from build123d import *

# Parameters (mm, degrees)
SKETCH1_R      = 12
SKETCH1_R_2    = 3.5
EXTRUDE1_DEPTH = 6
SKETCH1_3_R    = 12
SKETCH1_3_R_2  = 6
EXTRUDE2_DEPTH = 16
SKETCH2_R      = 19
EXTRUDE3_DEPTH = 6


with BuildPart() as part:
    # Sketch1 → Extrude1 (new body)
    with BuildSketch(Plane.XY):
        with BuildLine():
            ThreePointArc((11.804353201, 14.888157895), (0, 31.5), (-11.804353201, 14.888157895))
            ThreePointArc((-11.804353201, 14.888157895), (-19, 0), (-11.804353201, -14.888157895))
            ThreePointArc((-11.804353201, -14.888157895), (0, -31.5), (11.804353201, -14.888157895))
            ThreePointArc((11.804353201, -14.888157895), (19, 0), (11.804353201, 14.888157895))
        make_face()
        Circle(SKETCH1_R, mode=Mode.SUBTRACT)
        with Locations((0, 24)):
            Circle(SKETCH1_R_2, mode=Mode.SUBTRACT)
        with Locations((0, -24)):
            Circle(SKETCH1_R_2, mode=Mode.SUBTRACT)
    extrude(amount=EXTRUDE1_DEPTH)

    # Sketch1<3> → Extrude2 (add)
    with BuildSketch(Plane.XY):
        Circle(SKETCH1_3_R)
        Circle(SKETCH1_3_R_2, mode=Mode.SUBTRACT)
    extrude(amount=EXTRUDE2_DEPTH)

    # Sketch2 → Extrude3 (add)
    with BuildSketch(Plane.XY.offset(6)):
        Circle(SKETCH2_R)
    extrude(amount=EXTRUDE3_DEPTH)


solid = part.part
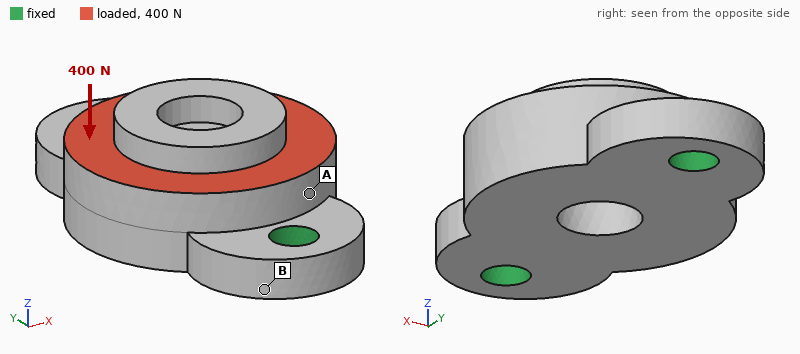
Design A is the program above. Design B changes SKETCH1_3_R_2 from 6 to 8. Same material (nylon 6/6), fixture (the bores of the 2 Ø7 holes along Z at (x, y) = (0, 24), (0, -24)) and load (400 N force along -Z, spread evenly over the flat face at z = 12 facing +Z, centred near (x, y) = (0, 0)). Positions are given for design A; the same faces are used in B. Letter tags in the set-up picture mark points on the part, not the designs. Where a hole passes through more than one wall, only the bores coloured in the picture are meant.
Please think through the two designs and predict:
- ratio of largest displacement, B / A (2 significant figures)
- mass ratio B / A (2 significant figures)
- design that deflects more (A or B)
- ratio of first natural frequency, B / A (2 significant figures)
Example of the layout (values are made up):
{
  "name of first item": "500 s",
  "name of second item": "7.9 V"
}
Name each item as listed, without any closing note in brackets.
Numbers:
{
  "ratio of largest displacement, B / A": "1.1",
  "mass ratio B / A": "0.95",
  "design that deflects more": "B",
  "ratio of first natural frequency, B / A": "1.0"
}
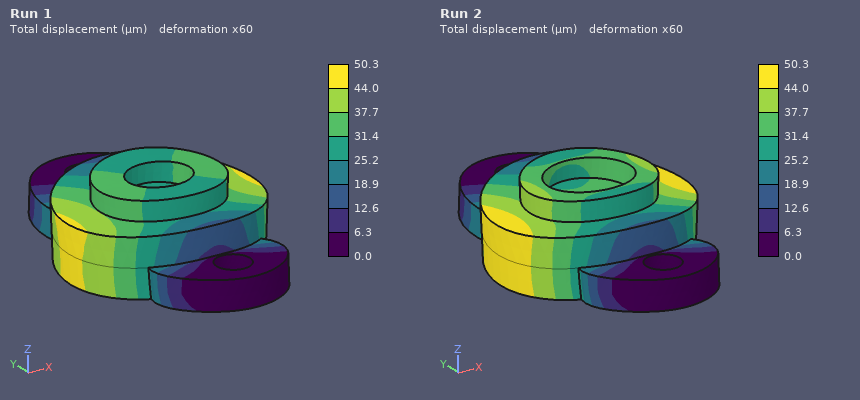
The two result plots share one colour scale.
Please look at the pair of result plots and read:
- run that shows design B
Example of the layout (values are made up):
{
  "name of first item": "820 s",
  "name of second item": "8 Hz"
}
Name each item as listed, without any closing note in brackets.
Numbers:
{
  "run that shows design B": "Run 2"
}
